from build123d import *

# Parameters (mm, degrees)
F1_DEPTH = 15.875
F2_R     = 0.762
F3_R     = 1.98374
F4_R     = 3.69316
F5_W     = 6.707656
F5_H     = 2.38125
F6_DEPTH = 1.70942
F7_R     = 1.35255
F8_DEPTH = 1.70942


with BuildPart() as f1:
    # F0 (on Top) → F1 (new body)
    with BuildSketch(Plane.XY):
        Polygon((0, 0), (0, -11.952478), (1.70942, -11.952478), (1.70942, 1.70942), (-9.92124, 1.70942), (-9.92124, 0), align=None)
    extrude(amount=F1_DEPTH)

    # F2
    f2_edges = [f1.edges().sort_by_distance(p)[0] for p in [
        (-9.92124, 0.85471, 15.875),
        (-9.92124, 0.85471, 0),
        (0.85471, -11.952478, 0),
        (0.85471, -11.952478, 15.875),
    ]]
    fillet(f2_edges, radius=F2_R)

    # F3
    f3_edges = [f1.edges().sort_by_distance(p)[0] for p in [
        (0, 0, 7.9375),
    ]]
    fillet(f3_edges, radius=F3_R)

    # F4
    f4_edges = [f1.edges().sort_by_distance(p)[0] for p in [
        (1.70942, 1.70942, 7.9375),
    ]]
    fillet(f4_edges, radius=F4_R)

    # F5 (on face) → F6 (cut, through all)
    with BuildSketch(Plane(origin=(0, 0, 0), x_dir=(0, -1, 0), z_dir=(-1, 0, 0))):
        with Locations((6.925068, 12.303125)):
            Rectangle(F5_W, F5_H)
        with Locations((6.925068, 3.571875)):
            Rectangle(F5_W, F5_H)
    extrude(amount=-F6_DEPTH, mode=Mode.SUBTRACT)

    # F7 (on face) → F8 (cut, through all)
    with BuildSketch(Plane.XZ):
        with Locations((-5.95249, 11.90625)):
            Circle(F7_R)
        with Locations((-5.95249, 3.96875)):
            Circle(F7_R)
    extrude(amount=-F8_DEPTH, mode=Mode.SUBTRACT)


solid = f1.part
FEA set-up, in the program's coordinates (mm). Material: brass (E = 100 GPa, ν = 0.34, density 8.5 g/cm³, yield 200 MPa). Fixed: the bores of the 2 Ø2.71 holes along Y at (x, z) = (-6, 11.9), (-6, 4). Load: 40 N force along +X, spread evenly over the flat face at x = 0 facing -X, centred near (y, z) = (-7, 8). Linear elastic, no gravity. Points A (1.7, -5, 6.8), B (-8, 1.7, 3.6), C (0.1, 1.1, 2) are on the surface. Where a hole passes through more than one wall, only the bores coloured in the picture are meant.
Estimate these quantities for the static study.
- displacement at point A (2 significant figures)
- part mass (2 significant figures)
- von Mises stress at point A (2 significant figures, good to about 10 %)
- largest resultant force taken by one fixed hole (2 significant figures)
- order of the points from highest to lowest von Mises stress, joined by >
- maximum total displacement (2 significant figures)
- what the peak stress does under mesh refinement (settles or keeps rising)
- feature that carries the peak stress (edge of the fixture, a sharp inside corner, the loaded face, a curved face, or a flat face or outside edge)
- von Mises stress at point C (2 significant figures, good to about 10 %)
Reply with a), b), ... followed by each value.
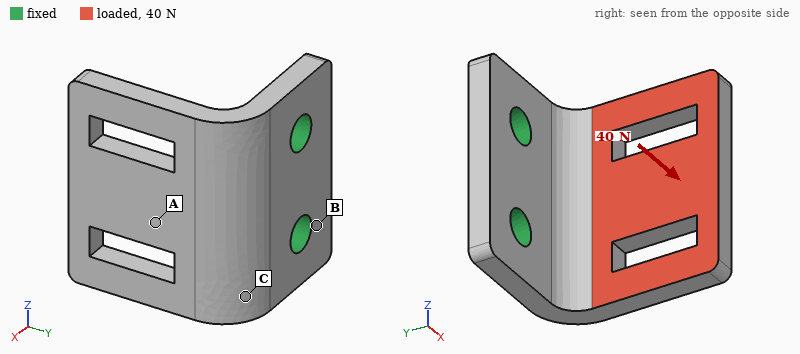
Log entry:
a) 22 µm
b) 4.5 g
c) 17 MPa
d) 21 N
e) C > A > B
f) 50 µm
g) keeps rising
h) edge of the fixture
i) 26 MPa
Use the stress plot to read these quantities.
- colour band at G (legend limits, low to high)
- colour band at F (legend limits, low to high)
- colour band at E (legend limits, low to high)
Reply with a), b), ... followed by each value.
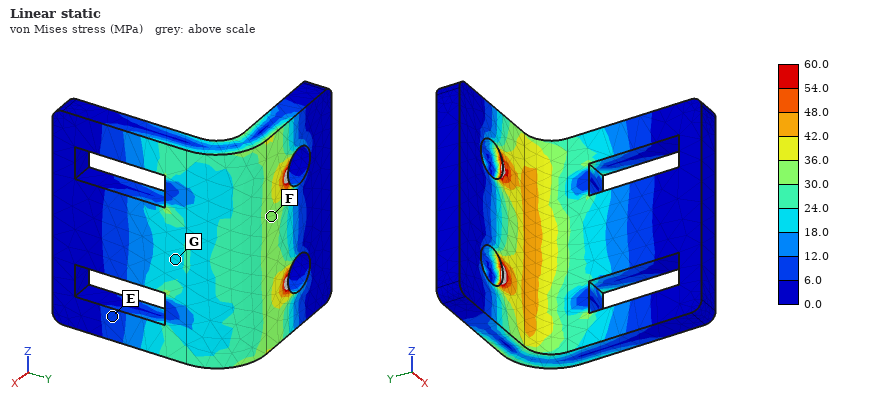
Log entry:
a) 18.0 to 24.0 MPa
b) 30.0 to 36.0 MPa
c) 6.0 to 12.0 MPa
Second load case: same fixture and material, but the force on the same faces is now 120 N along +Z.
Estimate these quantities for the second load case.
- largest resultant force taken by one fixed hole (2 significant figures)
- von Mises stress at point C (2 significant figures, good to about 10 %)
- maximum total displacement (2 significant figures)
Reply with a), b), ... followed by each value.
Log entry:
a) 130 N
b) 31 MPa
c) 41 µm
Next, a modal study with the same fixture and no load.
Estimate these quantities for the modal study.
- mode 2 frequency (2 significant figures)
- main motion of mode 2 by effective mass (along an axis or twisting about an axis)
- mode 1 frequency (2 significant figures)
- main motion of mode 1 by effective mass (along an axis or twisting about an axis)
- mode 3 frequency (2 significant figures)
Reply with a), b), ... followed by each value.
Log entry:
a) 7100 Hz
b) along Z
c) 3900 Hz
d) along X
e) 12 kHz
